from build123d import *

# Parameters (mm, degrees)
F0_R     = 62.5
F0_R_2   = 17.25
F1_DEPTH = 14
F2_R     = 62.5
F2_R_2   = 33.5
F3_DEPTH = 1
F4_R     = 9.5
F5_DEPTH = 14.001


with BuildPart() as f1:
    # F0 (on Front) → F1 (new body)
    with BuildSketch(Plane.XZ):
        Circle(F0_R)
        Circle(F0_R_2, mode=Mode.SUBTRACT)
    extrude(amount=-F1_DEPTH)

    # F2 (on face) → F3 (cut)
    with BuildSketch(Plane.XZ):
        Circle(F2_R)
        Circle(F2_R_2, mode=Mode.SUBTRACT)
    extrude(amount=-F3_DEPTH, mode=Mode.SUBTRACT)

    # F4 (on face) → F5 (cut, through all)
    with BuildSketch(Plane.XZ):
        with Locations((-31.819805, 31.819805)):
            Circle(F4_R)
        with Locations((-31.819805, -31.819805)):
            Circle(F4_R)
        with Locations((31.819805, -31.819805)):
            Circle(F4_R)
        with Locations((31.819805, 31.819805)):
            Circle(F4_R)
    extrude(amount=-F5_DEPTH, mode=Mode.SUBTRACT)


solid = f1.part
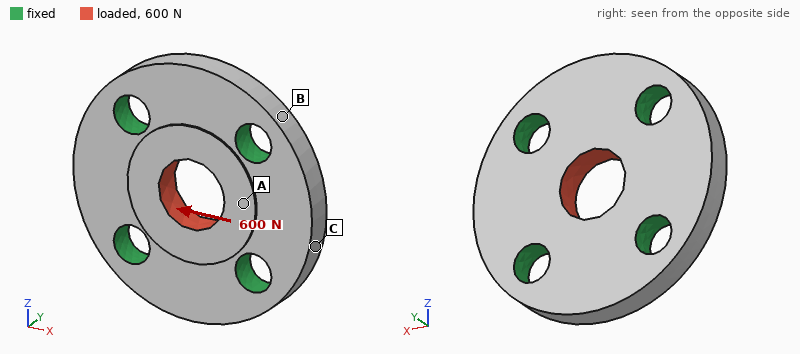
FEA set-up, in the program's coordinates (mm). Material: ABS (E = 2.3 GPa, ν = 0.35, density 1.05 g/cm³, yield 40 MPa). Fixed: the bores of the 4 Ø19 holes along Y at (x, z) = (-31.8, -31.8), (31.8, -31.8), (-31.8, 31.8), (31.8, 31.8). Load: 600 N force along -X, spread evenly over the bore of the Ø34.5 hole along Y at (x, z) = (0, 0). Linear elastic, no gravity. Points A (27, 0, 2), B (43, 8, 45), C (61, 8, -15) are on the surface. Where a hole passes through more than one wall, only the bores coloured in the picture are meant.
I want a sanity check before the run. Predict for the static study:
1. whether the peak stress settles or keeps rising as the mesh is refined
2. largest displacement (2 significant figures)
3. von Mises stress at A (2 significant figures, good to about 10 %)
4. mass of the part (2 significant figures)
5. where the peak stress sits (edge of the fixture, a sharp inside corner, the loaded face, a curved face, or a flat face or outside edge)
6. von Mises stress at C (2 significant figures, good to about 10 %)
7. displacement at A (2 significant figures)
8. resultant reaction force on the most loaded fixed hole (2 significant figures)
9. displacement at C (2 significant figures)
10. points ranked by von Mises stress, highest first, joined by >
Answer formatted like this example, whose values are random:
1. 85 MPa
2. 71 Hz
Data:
1. keeps rising
2. 6.4 µm
3. 0.26 MPa
4. 140 g
5. edge of the fixture
6. 0.14 MPa
7. 5.0 µm
8. 160 N
9. 2.2 µm
10. A > C > B
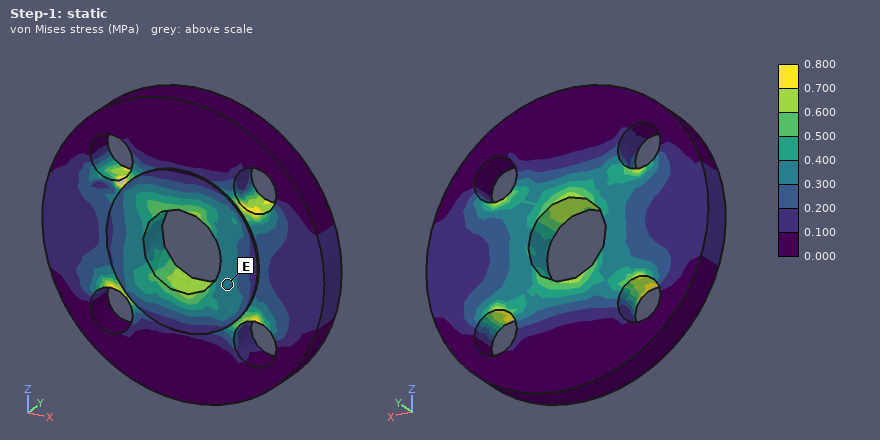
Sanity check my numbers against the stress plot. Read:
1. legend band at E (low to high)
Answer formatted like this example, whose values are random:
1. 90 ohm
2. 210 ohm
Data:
1. 0.300 to 0.400 MPa
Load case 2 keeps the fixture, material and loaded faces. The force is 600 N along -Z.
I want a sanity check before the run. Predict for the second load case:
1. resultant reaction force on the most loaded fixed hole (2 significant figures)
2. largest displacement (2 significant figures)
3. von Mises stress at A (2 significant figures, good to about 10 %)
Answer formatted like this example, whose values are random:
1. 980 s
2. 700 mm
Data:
1. 160 N
2. 6.4 µm
3. 0.24 MPa
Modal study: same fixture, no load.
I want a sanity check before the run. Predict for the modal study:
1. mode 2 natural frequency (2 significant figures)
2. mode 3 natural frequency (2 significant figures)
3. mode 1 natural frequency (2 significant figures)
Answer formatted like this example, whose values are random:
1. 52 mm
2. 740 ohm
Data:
1. 3800 Hz
2. 3800 Hz
3. 3700 Hz
